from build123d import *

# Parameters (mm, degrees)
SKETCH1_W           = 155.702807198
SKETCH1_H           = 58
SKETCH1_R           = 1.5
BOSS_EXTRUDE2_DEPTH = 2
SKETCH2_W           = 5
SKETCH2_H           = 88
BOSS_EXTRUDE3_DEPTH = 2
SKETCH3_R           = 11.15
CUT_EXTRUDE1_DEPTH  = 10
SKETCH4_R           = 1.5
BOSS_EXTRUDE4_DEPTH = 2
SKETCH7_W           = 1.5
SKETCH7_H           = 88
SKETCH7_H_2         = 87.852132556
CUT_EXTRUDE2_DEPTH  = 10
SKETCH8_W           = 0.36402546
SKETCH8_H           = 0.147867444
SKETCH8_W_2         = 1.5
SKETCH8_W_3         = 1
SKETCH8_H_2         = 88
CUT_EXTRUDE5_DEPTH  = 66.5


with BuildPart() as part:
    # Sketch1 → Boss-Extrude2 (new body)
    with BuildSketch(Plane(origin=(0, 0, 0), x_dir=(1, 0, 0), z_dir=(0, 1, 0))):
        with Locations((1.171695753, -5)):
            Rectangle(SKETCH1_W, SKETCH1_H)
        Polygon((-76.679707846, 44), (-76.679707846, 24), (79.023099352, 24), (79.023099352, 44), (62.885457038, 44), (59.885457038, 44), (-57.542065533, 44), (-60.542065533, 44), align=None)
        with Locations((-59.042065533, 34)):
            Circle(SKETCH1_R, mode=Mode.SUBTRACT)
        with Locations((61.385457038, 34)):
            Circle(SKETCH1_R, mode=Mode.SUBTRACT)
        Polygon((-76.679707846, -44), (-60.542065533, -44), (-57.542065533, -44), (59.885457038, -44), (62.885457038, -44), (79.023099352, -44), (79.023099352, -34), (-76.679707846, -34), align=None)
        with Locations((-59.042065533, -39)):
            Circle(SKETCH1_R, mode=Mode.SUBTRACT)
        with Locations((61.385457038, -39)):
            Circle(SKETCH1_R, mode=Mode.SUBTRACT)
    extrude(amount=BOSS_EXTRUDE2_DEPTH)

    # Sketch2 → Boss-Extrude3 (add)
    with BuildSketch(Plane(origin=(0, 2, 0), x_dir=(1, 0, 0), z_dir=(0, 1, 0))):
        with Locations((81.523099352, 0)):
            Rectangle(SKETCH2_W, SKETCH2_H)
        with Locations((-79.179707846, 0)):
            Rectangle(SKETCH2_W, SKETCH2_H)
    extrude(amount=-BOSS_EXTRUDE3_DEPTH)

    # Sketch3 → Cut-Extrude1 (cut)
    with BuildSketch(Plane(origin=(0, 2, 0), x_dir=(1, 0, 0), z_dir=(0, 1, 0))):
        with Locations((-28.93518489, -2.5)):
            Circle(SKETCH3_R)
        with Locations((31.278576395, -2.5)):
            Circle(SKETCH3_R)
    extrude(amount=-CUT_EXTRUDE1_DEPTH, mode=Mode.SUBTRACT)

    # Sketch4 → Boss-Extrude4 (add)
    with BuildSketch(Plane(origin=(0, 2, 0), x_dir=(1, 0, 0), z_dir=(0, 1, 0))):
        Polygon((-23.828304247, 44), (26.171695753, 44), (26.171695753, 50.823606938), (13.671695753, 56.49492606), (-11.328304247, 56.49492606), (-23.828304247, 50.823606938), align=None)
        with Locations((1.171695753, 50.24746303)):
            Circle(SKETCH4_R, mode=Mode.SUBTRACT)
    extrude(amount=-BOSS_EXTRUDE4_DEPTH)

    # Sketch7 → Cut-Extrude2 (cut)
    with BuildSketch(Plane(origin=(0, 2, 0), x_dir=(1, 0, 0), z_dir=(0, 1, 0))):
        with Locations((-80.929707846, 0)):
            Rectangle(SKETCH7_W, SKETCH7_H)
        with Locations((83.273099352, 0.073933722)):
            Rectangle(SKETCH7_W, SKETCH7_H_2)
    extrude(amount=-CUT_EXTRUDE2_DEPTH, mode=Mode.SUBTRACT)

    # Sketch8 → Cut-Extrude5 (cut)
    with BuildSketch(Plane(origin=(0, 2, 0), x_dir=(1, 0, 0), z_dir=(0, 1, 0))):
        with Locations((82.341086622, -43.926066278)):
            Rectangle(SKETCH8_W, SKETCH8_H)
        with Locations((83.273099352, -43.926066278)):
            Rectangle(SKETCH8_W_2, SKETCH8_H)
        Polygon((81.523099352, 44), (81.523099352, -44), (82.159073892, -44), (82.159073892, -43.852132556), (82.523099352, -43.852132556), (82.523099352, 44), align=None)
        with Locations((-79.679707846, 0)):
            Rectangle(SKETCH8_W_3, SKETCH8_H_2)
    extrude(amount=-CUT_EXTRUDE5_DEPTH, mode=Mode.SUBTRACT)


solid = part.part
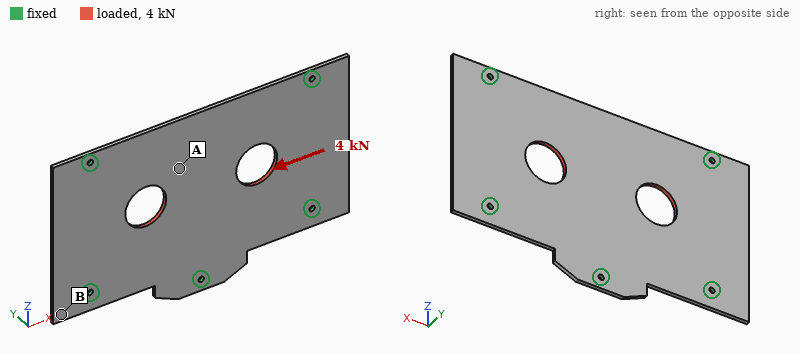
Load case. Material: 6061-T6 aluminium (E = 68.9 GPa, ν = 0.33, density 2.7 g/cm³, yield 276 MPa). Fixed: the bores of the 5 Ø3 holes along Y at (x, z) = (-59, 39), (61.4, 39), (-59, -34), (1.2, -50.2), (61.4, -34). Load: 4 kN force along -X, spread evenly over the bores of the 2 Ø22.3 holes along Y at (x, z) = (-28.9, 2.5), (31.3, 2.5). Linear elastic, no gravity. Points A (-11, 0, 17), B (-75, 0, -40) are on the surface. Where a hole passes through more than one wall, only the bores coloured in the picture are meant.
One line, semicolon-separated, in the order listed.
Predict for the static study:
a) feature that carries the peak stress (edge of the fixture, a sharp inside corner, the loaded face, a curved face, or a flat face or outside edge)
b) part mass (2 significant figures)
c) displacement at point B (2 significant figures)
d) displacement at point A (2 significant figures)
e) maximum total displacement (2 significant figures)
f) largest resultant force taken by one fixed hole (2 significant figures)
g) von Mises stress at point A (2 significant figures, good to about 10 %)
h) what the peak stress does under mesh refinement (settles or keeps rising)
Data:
edge of the fixture; 75 g; 3.7 µm; 14 µm; 17 µm; 910 N; 12 MPa; keeps rising
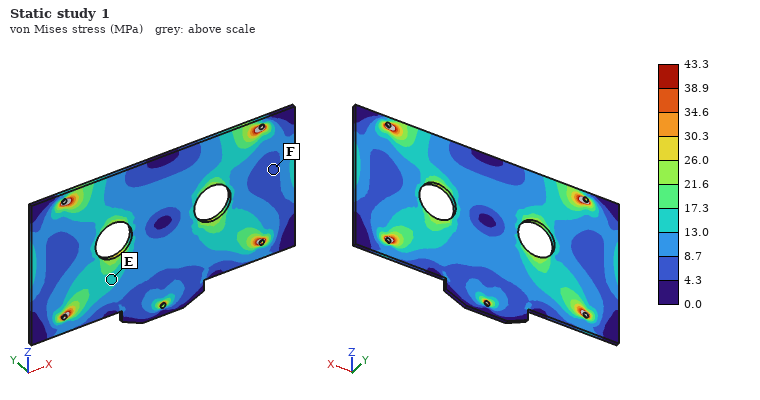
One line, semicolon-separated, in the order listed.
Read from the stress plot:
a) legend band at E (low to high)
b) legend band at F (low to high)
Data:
13.0 to 17.3 MPa; 4.3 to 8.7 MPa
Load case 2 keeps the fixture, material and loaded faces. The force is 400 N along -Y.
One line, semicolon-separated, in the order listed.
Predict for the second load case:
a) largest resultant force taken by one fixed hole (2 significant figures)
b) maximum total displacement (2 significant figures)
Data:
95 N; 0.72 mm
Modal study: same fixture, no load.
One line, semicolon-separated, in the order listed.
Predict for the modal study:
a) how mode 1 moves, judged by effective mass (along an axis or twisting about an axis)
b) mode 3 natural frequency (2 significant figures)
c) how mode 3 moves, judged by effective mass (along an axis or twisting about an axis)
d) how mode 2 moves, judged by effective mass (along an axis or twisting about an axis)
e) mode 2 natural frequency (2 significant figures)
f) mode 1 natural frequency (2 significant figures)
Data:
along Y; 1600 Hz; twisting about Z; along Y; 1400 Hz; 700 Hz
